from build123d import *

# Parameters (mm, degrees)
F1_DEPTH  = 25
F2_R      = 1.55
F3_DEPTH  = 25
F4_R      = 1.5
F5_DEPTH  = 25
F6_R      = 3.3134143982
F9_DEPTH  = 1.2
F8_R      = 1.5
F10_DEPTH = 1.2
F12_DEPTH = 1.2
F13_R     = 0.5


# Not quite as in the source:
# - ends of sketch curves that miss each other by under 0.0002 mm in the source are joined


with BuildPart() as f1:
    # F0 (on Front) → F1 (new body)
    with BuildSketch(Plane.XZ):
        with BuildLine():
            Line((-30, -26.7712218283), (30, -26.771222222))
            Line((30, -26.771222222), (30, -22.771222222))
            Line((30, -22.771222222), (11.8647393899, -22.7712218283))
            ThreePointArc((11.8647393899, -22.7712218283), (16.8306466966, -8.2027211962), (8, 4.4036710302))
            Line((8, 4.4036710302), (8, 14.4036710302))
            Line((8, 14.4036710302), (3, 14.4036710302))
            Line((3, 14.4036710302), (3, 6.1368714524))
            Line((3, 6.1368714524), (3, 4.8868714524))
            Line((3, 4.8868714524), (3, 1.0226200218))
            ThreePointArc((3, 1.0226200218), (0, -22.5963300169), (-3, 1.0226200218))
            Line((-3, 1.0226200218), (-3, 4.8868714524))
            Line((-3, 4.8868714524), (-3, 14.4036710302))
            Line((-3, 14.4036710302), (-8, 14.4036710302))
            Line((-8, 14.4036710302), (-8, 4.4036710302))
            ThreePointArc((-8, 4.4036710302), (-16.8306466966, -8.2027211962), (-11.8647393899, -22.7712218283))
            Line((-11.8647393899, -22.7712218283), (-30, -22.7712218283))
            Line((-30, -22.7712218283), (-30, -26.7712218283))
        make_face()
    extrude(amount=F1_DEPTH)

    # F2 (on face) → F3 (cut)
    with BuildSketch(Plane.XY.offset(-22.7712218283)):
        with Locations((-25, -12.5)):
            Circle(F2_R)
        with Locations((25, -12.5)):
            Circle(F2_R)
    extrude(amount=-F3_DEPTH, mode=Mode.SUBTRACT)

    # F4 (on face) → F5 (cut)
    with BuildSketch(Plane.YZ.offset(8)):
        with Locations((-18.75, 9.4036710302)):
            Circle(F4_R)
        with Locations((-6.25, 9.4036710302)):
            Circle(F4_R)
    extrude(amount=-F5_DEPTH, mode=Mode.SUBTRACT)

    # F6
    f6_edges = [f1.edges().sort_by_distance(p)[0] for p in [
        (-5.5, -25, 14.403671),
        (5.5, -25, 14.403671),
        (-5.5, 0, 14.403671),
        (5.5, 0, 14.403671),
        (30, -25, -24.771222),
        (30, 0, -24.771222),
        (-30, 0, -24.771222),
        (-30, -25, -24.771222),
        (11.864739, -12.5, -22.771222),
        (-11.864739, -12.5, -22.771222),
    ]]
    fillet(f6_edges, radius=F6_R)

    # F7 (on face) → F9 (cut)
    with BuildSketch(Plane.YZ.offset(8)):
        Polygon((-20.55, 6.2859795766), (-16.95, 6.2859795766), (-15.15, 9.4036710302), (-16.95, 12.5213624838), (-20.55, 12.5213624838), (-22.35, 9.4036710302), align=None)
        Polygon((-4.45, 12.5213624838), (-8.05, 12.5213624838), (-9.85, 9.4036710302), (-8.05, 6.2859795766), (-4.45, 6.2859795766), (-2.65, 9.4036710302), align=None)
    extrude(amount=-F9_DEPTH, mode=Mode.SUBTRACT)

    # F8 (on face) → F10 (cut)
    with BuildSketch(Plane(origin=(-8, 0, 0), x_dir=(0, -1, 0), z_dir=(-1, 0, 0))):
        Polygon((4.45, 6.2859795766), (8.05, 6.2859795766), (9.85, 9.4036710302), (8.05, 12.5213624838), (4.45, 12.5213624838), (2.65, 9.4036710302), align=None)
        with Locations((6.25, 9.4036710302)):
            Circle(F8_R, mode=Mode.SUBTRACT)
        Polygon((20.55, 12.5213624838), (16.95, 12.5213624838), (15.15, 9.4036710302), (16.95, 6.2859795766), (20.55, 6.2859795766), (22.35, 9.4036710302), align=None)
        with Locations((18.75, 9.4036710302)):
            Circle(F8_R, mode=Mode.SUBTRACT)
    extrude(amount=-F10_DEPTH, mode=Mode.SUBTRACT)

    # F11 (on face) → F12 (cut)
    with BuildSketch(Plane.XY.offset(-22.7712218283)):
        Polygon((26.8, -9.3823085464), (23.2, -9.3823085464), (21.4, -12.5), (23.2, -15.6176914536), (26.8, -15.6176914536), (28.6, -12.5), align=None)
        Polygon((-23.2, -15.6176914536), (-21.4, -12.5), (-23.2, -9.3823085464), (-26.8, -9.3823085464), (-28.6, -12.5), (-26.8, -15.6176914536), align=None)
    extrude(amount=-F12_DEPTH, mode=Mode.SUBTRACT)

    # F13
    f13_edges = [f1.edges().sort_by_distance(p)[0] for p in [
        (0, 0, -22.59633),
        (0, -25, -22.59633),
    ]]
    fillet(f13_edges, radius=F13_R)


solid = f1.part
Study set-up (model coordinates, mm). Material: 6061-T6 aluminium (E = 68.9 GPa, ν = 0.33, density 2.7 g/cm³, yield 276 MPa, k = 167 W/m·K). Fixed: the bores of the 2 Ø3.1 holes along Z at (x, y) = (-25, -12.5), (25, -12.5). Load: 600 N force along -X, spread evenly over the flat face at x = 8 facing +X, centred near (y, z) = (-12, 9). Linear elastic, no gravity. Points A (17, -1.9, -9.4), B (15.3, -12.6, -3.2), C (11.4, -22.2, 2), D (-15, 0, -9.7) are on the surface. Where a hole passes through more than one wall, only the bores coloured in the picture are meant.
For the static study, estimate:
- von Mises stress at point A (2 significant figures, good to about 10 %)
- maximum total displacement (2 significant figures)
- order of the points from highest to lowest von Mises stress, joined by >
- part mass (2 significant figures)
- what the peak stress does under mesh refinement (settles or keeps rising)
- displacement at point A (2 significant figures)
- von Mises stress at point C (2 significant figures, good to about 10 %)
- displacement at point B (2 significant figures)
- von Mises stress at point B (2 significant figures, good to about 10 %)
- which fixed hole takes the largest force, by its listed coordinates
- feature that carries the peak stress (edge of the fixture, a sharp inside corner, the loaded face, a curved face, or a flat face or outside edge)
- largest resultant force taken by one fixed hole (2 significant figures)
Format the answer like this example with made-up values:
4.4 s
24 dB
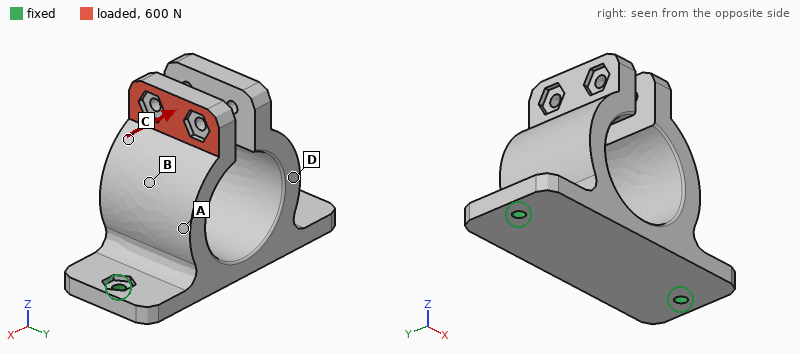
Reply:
100 MPa
0.60 mm
A > B > C > D
45 g
keeps rising
0.12 mm
50 MPa
0.22 mm
65 MPa
(-25, -12.5)
edge of the fixture
890 N
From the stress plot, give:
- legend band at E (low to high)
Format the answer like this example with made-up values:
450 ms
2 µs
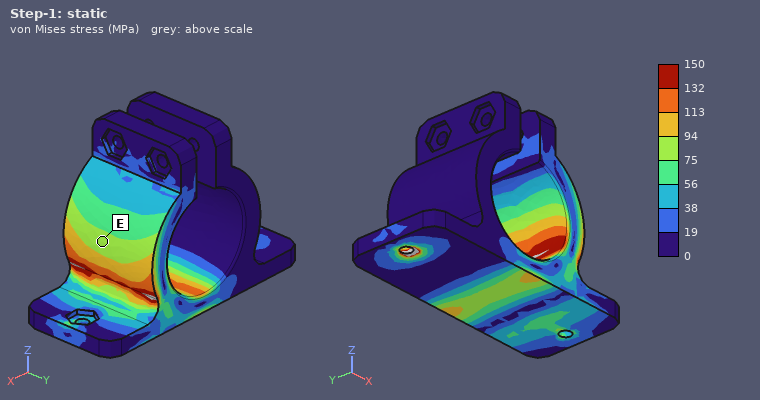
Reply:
75 to 94 MPa
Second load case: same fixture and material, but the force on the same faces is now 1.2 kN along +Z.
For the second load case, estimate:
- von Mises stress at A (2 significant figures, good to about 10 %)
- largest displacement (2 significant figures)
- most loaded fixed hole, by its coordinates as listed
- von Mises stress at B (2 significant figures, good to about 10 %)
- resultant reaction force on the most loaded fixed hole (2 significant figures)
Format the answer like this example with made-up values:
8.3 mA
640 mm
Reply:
59 MPa
0.33 mm
(25, -12.5)
38 MPa
1.1 kN
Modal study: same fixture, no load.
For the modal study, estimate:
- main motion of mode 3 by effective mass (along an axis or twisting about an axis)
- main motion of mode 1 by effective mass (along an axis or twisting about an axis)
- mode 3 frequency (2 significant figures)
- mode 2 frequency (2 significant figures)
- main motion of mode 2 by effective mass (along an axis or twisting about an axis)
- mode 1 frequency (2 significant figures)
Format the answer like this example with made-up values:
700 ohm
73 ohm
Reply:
along X
along Y
2900 Hz
2000 Hz
along Z
1600 Hz
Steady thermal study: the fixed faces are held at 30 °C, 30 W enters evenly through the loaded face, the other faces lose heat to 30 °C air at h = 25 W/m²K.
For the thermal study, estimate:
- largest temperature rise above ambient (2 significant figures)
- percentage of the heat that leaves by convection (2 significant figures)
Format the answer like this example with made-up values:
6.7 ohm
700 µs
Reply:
66 K
13 %
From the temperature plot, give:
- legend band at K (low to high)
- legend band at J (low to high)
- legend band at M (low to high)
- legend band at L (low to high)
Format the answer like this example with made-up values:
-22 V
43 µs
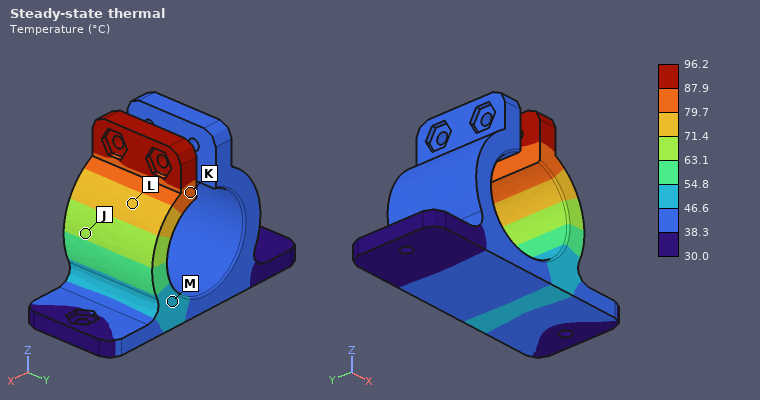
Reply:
79.7 to 87.9 °C
63.1 to 71.4 °C
46.6 to 54.8 °C
71.4 to 79.7 °C
